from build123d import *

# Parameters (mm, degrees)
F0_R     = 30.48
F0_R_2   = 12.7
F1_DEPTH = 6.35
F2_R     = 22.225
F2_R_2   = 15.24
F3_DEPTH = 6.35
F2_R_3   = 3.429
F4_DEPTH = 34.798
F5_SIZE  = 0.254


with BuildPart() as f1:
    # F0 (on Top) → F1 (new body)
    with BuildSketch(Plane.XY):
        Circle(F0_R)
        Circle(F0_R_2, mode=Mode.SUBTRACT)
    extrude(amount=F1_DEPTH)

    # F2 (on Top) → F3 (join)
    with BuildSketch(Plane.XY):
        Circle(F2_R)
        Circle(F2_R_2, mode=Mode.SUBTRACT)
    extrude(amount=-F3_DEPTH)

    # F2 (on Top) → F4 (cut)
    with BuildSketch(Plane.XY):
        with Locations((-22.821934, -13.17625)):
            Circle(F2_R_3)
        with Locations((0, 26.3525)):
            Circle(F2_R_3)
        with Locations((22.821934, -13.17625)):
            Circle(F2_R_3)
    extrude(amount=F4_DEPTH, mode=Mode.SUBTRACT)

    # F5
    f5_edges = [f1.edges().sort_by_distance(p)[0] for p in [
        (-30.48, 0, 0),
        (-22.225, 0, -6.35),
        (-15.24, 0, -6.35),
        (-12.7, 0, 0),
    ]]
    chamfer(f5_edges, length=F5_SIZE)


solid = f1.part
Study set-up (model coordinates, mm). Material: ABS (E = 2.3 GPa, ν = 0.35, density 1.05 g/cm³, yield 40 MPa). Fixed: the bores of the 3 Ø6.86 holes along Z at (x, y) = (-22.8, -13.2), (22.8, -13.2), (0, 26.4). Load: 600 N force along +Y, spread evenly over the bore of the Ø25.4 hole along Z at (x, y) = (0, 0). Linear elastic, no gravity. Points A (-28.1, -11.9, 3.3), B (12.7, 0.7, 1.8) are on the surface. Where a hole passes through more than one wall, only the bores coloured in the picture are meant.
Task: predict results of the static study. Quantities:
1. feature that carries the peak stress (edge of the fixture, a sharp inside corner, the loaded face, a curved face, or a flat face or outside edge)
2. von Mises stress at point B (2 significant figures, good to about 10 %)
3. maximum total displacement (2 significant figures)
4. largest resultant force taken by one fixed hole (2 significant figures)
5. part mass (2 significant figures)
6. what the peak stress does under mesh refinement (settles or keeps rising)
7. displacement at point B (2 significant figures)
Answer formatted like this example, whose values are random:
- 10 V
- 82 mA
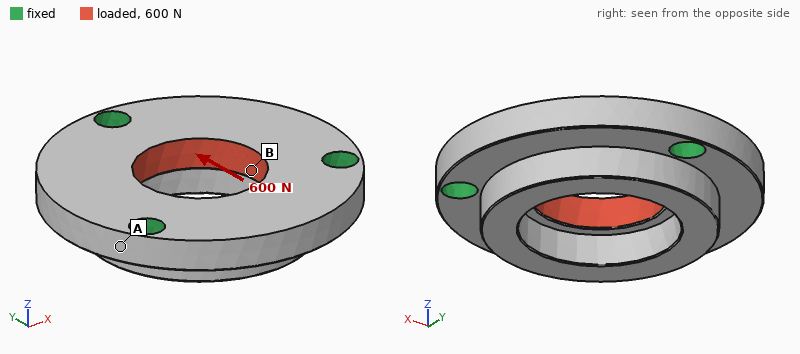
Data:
- edge of the fixture
- 2.2 MPa
- 28 µm
- 220 N
- 21 g
- keeps rising
- 16 µm
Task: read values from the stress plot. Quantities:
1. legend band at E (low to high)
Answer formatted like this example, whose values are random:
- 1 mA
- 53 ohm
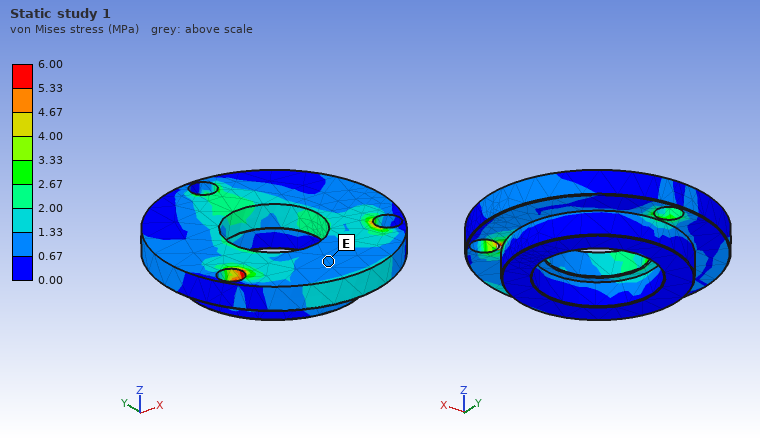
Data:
- 0.67 to 1.33 MPa
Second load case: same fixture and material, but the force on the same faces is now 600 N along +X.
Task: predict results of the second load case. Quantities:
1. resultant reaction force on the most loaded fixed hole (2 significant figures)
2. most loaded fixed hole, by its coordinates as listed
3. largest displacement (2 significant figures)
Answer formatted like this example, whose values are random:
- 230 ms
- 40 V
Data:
- 230 N
- (0, 26.4)
- 25 µm
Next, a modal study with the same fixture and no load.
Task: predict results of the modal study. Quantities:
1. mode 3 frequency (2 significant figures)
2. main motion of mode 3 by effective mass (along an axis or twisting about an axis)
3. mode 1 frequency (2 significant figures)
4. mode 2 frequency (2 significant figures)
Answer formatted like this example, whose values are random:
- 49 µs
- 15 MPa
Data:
- 4700 Hz
- along Z
- 3800 Hz
- 3800 Hz
